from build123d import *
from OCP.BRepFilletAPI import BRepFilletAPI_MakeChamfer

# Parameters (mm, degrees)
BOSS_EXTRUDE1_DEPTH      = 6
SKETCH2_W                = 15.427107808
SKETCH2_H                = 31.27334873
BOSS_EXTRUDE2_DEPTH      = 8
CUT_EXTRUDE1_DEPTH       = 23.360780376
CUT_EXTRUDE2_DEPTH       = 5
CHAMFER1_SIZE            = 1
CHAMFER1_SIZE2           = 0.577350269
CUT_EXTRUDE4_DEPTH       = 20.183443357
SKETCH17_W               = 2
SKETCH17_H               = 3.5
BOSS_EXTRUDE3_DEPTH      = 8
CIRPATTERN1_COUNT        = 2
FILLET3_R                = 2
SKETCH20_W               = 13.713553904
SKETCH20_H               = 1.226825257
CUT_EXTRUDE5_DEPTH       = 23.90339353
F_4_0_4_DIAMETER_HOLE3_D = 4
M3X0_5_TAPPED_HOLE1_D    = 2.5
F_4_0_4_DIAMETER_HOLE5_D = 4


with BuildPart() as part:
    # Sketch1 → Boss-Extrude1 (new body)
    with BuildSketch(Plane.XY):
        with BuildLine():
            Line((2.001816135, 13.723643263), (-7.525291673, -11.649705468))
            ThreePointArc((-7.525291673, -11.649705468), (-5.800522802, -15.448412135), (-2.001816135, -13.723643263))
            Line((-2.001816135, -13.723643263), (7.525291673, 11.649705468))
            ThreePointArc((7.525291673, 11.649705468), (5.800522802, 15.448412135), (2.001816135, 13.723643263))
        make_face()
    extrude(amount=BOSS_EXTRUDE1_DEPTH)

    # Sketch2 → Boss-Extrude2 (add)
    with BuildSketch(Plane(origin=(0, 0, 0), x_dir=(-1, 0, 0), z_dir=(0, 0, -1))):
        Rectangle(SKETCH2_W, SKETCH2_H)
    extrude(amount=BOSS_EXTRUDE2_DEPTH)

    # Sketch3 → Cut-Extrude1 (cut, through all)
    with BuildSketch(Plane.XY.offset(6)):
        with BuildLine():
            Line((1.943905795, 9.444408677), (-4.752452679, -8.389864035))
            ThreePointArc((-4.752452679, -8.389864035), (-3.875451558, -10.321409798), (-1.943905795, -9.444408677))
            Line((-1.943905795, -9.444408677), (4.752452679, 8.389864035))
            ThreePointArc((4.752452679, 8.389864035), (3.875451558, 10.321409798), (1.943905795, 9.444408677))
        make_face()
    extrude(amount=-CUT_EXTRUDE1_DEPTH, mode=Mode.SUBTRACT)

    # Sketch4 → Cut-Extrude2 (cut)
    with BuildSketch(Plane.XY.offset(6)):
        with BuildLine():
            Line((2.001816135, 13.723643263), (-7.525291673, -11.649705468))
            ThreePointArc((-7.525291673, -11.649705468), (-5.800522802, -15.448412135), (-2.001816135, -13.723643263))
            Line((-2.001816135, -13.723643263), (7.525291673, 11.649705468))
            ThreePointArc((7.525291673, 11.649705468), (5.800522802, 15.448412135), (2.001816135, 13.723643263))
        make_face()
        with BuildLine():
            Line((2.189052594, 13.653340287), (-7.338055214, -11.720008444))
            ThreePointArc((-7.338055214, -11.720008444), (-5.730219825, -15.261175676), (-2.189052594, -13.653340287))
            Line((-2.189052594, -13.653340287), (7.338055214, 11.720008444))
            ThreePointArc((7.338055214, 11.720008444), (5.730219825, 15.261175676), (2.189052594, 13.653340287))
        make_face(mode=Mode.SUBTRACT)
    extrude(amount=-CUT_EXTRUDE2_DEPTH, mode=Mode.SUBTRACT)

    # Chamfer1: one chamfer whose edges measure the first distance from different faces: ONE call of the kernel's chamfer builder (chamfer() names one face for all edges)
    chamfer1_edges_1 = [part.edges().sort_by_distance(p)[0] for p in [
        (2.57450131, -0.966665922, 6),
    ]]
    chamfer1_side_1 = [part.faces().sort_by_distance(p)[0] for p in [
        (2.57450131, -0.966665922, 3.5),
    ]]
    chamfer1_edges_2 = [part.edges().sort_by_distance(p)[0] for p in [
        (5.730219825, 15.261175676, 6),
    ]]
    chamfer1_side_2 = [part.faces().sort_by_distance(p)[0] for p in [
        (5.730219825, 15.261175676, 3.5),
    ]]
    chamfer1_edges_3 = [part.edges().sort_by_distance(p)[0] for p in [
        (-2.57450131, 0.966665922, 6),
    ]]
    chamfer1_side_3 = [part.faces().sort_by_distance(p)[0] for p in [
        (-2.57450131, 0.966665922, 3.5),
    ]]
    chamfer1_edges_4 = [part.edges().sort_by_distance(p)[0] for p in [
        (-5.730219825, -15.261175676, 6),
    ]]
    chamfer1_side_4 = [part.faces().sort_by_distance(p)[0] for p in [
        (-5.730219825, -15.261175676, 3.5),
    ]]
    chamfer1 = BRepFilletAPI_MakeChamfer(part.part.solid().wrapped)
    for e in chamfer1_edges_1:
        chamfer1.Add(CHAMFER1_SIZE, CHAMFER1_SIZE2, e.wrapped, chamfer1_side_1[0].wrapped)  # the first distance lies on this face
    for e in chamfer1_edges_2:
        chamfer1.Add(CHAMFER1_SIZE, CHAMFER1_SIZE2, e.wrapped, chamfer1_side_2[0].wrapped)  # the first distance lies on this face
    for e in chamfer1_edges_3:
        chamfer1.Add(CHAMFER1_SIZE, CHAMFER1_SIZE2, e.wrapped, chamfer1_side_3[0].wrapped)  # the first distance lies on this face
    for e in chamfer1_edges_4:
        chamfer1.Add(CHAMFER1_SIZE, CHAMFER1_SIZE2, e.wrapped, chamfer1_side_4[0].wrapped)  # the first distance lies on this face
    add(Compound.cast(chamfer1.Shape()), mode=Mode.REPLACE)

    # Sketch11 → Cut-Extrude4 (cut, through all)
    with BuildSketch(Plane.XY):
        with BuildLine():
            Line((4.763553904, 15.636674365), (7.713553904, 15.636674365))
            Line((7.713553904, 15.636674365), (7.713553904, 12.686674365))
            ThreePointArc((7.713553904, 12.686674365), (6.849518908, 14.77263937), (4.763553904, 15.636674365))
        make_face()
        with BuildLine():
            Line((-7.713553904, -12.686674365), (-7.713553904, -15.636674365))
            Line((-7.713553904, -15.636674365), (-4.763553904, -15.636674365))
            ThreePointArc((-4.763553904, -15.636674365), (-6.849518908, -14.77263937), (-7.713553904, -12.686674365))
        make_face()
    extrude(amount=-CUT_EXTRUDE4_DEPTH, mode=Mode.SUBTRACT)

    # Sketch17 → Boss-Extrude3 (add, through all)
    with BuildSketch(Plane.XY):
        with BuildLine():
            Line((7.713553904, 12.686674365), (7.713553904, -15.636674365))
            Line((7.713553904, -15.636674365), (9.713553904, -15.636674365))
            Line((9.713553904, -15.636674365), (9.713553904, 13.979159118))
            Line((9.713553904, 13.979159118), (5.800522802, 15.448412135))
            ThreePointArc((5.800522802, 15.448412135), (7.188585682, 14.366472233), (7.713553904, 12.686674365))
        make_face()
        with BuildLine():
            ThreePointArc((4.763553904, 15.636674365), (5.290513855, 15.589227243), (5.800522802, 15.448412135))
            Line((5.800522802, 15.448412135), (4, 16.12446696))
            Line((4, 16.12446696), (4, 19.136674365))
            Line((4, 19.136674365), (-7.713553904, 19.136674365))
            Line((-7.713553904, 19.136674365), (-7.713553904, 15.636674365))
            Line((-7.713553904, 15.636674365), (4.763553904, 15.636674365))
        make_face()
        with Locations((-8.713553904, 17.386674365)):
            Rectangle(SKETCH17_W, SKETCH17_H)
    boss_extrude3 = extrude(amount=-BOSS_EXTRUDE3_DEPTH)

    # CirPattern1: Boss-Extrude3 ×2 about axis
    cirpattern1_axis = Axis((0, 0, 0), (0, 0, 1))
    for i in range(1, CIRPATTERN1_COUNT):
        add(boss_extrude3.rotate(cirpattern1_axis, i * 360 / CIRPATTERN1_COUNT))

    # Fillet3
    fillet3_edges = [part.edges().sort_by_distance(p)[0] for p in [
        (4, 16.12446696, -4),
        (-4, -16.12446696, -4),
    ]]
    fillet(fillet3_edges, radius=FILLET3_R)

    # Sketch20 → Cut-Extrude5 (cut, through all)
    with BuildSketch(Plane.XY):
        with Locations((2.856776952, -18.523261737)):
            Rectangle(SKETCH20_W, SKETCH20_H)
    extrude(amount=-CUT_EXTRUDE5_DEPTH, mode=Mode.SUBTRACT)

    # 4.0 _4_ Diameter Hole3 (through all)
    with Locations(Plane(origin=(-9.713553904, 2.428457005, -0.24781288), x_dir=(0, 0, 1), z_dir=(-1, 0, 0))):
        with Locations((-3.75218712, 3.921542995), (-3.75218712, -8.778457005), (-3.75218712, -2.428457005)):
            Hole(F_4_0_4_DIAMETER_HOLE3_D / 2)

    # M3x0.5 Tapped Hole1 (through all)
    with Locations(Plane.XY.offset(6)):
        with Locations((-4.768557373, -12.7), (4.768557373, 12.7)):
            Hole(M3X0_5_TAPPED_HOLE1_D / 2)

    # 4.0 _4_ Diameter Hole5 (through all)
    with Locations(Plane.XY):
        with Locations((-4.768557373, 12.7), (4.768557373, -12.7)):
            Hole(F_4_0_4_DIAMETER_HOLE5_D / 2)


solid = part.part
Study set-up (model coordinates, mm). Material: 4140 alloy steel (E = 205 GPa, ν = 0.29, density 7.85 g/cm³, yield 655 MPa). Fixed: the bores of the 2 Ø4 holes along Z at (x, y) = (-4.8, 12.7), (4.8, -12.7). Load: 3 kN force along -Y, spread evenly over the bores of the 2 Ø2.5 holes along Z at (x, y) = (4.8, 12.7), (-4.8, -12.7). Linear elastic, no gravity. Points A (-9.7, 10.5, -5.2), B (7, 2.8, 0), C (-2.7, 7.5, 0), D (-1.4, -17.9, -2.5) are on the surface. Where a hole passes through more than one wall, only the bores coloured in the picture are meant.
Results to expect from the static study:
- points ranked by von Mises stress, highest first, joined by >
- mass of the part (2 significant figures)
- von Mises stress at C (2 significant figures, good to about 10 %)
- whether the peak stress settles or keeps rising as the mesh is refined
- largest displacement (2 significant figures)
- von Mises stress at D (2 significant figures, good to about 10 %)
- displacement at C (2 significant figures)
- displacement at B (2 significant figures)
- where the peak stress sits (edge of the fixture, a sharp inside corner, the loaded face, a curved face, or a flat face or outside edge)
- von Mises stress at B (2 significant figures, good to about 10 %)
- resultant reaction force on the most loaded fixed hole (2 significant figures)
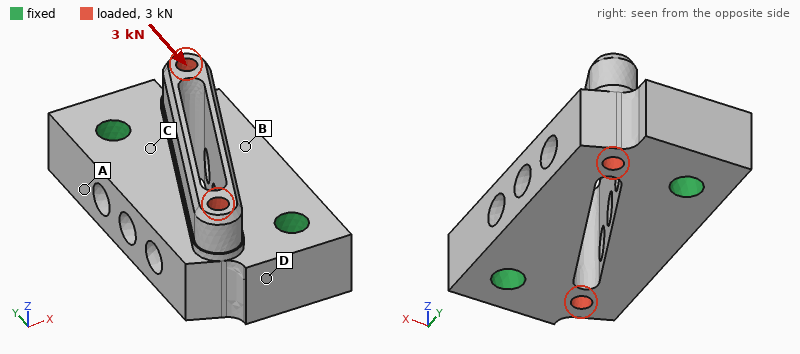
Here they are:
B > C > D > A
36 g
24 MPa
keeps rising
4.7 µm
15 MPa
1.1 µm
2.0 µm
edge of the fixture
33 MPa
1.5 kN
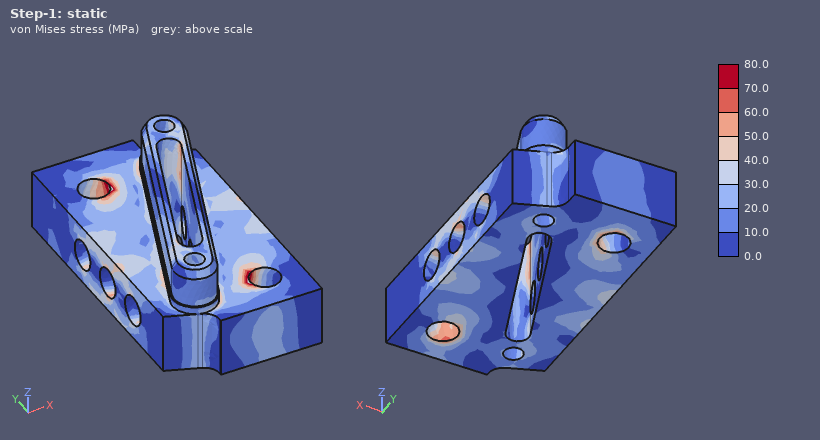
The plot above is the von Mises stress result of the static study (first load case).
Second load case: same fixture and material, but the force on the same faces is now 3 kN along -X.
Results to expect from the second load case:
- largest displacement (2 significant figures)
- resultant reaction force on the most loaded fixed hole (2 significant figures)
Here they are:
9.2 µm
1.5 kN
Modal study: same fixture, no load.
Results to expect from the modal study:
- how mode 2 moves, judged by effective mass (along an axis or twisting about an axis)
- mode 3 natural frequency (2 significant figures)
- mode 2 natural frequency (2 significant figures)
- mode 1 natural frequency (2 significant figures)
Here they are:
along Z
30 kHz
25 kHz
23 kHz
